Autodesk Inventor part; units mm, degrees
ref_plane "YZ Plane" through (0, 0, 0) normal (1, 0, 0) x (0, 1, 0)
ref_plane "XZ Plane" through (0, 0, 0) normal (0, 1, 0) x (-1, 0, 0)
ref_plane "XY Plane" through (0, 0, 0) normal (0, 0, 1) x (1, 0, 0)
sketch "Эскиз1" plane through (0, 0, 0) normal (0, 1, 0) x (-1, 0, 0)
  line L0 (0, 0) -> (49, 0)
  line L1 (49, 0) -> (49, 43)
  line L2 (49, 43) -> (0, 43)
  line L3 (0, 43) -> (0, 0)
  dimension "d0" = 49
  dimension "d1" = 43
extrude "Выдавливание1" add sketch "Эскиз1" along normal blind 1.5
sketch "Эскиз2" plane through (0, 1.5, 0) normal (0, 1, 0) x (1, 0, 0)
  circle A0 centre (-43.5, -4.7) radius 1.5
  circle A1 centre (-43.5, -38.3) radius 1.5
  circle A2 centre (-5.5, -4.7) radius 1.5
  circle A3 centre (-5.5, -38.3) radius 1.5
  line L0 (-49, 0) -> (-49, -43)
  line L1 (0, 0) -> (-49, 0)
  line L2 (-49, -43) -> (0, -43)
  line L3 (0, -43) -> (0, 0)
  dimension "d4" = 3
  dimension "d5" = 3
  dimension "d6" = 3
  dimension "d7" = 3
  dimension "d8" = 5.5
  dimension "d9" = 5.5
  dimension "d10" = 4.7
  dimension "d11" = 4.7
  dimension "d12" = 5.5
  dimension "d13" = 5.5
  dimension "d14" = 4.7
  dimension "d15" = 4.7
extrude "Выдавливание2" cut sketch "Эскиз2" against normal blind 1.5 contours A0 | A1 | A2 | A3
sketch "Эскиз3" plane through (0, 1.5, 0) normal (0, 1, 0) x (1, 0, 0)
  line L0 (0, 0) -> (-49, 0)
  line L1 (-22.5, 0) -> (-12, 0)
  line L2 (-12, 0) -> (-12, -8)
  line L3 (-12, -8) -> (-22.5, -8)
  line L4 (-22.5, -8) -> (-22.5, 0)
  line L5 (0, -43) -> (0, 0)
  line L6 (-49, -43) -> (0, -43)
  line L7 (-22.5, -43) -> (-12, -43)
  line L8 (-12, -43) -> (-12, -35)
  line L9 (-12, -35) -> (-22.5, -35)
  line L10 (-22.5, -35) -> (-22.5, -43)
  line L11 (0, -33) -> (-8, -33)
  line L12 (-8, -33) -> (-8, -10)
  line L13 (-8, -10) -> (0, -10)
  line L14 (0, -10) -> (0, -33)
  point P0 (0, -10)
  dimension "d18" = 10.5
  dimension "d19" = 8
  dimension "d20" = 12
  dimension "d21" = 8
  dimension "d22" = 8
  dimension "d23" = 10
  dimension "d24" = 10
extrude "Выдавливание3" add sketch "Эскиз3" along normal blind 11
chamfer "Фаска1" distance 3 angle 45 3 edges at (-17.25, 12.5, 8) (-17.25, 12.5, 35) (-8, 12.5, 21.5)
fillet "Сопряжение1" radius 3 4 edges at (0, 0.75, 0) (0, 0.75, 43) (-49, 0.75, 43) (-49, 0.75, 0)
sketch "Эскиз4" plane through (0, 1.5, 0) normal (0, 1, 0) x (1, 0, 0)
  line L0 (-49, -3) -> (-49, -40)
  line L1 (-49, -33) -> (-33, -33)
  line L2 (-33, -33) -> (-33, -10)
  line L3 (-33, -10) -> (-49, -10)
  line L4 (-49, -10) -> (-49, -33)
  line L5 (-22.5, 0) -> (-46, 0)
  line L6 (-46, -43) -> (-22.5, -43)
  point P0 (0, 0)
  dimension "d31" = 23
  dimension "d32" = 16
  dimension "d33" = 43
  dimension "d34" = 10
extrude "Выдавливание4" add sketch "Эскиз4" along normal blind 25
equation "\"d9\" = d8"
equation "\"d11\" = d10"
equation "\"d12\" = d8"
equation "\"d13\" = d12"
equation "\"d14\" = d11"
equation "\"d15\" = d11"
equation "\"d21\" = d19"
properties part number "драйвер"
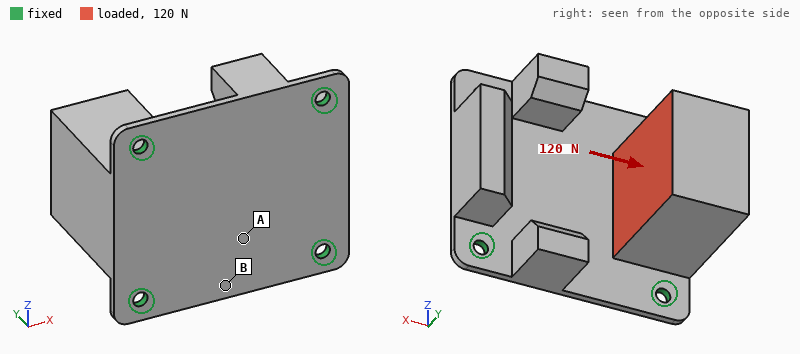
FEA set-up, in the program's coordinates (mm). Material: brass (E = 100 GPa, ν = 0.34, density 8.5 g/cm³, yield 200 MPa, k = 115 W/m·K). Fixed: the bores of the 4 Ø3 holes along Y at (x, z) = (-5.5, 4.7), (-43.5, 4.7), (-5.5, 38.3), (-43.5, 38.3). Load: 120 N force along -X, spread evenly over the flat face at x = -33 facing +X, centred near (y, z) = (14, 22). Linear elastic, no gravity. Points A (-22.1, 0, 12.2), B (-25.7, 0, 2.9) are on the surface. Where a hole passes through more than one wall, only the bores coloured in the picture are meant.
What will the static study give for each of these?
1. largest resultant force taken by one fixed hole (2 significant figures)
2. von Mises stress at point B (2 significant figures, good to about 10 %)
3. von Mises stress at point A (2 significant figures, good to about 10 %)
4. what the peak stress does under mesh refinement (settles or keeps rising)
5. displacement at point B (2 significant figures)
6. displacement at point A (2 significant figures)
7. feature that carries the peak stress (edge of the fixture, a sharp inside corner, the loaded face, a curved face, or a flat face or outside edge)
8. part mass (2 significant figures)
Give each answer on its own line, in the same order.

45 N
16 MPa
7.5 MPa
keeps rising
17 µm
19 µm
edge of the fixture
140 g
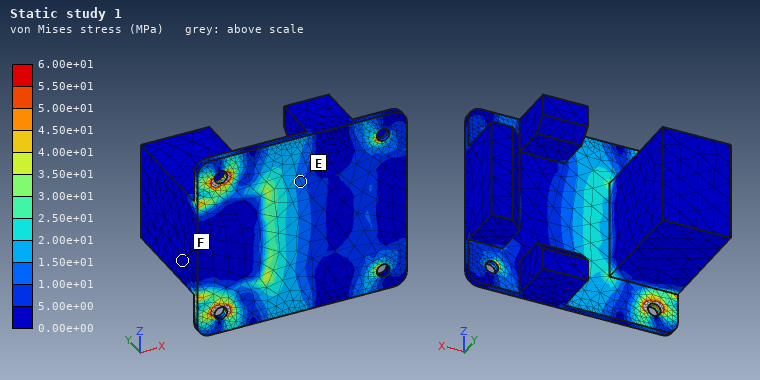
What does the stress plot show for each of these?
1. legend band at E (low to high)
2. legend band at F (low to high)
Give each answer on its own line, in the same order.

1.00e+01 to 1.50e+01 MPa
0.00e+00 to 5.00e+00 MPa
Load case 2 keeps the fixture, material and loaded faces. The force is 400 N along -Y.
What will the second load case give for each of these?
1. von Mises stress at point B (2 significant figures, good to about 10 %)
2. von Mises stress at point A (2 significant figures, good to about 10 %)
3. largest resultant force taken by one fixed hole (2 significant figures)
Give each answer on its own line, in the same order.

45 MPa
20 MPa
170 N
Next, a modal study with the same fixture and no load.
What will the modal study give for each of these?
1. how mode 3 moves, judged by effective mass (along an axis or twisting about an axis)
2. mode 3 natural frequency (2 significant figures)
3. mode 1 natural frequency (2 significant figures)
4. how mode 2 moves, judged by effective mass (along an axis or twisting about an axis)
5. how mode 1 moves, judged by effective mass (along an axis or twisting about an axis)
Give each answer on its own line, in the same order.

along Y
3000 Hz
950 Hz
along Z
along X
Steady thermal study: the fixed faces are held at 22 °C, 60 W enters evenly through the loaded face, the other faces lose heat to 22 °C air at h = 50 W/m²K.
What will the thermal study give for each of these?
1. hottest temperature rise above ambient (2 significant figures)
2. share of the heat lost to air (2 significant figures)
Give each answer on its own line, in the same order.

79 K
20 %
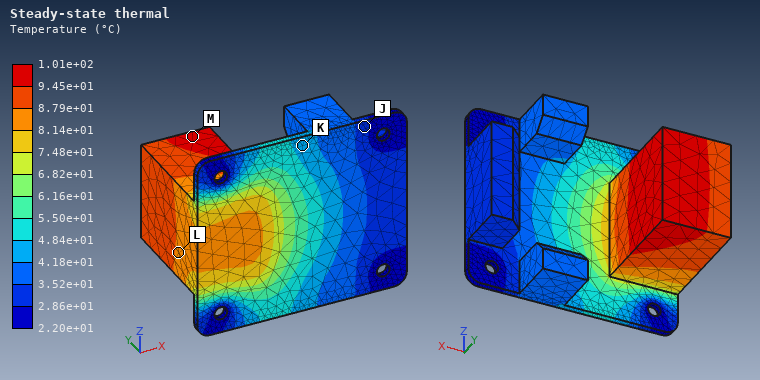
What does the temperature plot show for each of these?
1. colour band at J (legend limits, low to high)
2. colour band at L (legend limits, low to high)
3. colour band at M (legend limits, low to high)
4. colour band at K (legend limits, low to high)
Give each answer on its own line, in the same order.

2.86e+01 to 3.52e+01 °C
8.14e+01 to 8.79e+01 °C
9.45e+01 to 1.01e+02 °C
4.18e+01 to 4.84e+01 °C
